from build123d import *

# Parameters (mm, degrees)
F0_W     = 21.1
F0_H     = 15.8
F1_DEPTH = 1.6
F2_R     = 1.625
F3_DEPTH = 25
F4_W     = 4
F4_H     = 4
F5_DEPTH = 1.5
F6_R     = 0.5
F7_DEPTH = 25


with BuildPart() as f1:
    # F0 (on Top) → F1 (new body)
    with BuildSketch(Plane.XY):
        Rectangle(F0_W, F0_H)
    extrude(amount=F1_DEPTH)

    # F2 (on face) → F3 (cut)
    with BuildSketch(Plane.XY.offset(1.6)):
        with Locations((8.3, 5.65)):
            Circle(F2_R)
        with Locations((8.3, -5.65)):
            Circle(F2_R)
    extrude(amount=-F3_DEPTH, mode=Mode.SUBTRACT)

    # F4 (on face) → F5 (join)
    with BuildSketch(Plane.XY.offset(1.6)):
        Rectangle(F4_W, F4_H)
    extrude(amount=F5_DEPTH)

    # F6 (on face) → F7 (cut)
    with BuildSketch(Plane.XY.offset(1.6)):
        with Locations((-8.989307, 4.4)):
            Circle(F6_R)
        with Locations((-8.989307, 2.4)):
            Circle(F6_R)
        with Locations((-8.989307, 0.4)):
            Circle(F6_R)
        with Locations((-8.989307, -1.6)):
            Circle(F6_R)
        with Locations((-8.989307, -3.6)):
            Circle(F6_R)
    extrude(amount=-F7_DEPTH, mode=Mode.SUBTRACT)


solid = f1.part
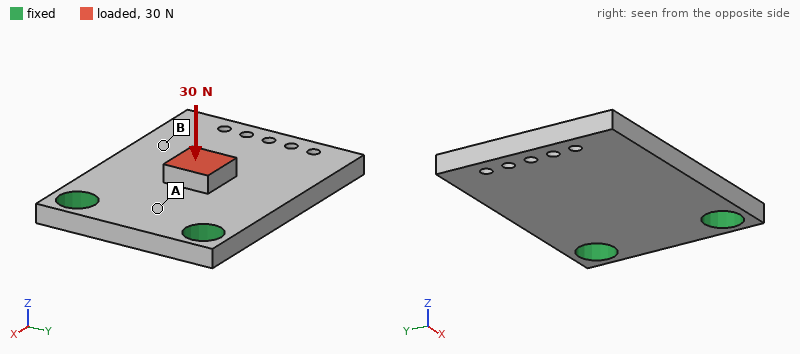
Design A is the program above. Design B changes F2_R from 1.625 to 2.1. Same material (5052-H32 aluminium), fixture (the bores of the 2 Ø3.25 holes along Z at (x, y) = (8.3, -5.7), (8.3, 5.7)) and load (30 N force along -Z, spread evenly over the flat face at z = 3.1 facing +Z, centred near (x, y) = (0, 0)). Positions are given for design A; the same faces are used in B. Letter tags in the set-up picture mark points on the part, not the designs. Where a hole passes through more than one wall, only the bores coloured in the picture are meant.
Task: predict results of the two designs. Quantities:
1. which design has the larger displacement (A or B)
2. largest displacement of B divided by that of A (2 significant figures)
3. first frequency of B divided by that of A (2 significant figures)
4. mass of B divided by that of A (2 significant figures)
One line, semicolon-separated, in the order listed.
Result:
A; 0.83; 1.1; 0.97
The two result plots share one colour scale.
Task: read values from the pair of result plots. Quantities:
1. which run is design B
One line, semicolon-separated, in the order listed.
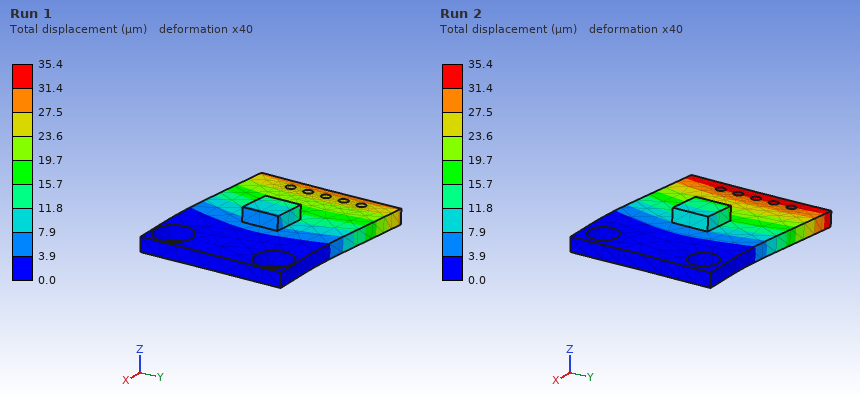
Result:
Run 1
